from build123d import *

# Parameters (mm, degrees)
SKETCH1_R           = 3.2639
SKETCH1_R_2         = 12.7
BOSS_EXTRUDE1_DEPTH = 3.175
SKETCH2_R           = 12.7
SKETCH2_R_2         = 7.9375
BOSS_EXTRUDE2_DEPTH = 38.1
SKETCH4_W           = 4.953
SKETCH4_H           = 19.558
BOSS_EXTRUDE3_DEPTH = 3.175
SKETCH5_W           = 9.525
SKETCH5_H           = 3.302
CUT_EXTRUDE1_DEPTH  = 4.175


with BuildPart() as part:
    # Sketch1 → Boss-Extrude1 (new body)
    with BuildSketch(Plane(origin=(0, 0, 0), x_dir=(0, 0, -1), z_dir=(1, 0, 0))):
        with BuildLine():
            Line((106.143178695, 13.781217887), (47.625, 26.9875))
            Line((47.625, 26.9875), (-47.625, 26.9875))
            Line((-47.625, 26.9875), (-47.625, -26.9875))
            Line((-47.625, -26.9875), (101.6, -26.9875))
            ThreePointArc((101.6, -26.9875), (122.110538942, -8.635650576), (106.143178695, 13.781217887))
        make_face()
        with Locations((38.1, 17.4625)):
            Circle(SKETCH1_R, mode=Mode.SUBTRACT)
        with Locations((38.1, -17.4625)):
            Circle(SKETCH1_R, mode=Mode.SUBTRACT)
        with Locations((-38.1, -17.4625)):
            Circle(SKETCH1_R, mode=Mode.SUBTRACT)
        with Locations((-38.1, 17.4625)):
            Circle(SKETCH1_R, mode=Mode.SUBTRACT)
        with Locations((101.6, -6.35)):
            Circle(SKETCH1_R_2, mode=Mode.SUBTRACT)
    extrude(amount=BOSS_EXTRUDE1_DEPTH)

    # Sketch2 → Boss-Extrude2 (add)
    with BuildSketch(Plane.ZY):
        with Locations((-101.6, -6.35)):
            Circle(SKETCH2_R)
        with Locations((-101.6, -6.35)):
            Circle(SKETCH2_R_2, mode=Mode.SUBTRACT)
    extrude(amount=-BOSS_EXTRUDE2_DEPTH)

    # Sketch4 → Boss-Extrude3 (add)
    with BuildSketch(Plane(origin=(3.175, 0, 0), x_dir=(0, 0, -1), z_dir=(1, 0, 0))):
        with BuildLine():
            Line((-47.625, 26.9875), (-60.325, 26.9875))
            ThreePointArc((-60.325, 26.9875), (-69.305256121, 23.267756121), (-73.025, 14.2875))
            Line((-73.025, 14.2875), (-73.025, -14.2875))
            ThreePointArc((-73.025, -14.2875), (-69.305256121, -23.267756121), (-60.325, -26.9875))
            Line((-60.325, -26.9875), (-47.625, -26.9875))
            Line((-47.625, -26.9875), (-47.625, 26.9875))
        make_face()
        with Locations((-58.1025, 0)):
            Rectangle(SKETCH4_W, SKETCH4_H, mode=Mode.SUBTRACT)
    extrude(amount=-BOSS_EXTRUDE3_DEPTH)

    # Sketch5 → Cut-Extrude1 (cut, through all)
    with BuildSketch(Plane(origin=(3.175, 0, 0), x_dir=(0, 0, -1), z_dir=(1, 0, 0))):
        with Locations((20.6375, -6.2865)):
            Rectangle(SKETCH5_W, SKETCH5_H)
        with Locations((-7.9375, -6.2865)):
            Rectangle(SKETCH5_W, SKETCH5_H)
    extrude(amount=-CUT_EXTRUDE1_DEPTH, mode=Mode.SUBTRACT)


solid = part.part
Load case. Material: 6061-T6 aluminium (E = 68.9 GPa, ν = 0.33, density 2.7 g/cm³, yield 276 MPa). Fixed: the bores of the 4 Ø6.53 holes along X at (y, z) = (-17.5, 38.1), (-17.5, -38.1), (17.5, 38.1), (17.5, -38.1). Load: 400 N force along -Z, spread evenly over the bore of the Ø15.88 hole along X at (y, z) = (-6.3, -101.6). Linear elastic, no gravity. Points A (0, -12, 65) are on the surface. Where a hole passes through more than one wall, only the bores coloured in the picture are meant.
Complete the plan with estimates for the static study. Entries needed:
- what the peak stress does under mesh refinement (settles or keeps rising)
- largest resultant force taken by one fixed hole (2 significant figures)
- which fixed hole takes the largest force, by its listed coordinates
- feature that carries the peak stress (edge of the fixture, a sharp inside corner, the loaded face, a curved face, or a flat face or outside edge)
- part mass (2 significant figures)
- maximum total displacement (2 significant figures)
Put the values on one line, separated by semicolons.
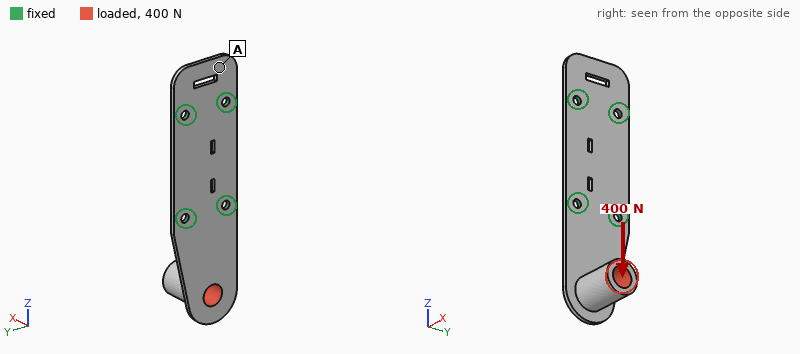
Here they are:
keeps rising; 250 N; (-17.5, -38.1); edge of the fixture; 110 g; 2.4 mm
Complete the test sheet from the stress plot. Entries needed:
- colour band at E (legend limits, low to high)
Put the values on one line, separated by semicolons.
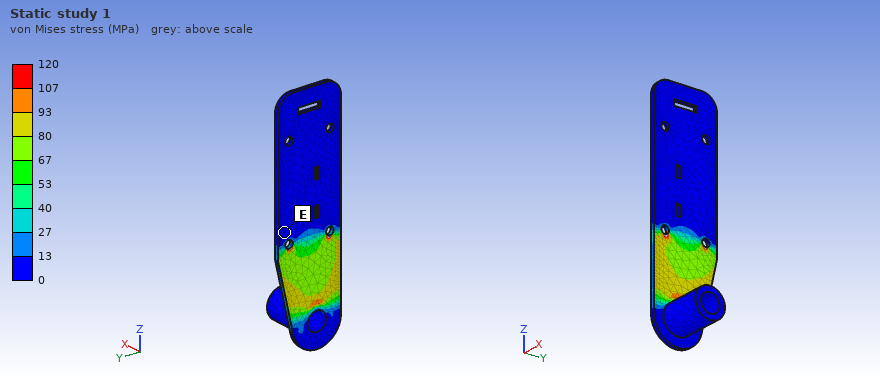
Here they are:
0 to 13 MPa
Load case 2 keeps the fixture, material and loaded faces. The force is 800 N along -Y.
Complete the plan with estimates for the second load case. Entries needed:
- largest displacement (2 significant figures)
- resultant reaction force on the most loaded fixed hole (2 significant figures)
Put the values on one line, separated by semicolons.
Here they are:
1.6 mm; 1.4 kN
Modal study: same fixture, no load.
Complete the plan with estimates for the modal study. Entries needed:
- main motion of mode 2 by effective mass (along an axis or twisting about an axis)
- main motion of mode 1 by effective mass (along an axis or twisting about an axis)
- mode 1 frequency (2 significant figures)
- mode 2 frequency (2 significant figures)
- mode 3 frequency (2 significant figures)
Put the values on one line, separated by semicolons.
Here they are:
along Y; along X; 250 Hz; 710 Hz; 1300 Hz
